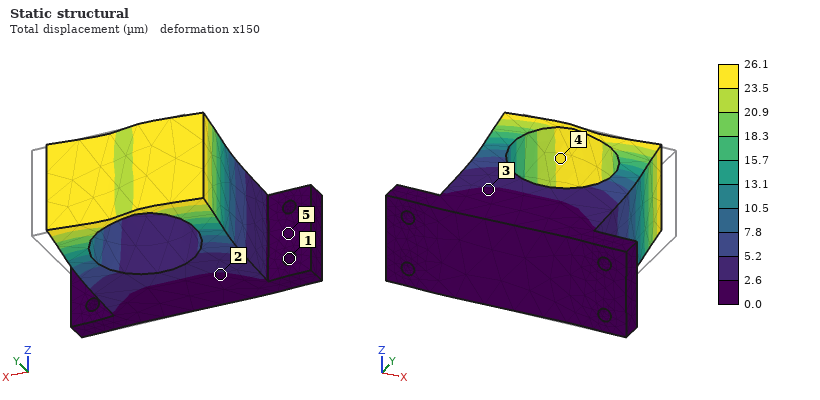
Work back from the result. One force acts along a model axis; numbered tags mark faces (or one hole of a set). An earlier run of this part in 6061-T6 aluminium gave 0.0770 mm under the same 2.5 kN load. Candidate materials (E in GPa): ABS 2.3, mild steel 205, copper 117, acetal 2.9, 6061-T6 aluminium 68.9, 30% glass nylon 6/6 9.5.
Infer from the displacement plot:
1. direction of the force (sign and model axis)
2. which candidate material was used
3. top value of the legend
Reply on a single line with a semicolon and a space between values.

-X; mild steel; 26.1 µm
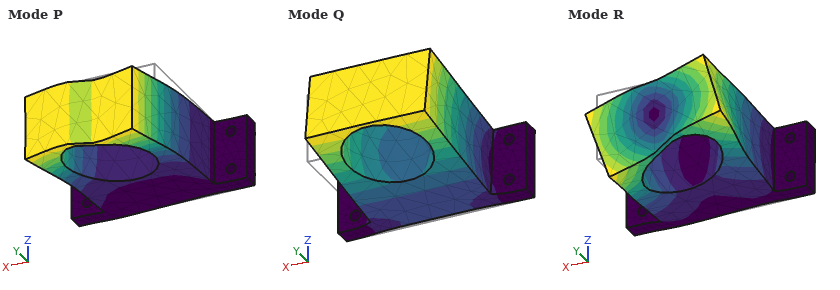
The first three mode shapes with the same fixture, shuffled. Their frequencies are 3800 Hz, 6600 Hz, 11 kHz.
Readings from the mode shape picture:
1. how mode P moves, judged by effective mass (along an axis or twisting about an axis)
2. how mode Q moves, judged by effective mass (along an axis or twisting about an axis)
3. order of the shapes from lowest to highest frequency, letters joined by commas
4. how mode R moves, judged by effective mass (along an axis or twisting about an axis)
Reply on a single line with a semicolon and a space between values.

along X; along Z; Q, P, R; twisting about Y
